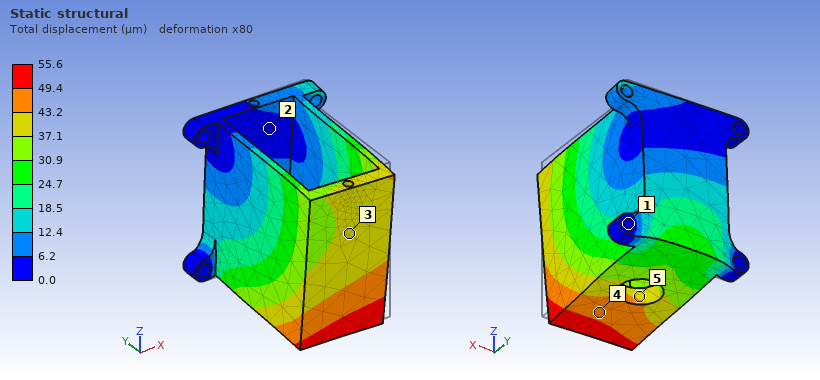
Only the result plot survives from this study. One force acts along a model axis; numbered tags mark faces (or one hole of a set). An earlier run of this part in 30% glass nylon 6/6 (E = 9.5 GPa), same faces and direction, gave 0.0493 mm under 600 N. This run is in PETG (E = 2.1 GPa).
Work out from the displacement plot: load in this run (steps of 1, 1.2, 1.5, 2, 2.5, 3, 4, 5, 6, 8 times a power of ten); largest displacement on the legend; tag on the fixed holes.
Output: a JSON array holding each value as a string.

["150 N", "55.6 µm", "1"]
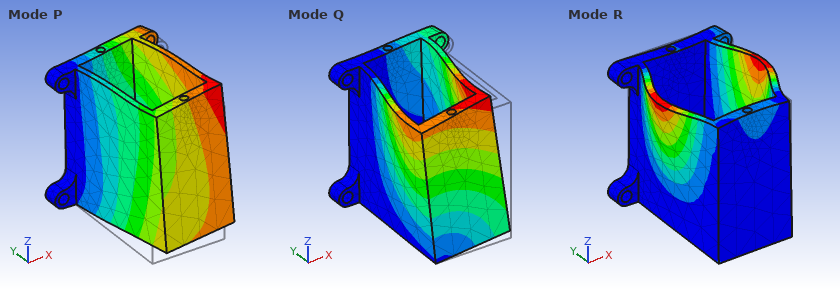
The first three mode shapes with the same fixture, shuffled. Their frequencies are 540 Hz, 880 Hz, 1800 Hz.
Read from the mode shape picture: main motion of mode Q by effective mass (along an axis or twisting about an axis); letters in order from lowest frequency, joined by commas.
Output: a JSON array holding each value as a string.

["along X", "Q, P, R"]
